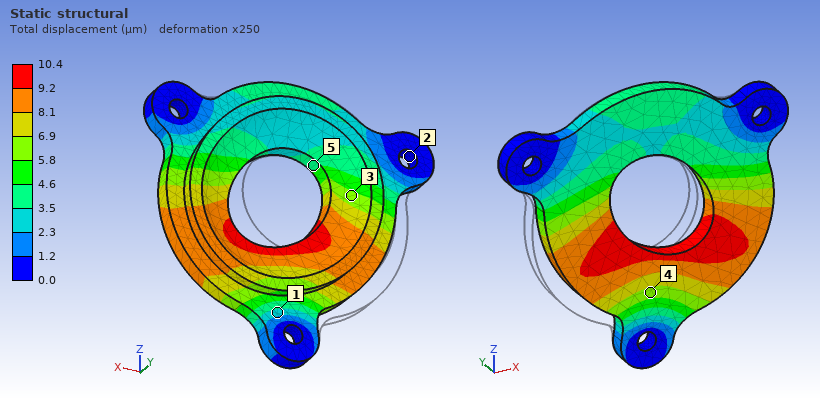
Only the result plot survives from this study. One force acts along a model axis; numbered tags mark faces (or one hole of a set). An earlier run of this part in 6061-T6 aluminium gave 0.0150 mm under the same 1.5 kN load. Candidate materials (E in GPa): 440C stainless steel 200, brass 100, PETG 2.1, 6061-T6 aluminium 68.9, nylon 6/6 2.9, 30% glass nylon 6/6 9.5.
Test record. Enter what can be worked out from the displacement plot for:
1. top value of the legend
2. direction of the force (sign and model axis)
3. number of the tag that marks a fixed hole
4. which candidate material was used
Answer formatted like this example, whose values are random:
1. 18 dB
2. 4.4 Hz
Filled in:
1. 10.4 µm
2. +X
3. 2
4. brass
